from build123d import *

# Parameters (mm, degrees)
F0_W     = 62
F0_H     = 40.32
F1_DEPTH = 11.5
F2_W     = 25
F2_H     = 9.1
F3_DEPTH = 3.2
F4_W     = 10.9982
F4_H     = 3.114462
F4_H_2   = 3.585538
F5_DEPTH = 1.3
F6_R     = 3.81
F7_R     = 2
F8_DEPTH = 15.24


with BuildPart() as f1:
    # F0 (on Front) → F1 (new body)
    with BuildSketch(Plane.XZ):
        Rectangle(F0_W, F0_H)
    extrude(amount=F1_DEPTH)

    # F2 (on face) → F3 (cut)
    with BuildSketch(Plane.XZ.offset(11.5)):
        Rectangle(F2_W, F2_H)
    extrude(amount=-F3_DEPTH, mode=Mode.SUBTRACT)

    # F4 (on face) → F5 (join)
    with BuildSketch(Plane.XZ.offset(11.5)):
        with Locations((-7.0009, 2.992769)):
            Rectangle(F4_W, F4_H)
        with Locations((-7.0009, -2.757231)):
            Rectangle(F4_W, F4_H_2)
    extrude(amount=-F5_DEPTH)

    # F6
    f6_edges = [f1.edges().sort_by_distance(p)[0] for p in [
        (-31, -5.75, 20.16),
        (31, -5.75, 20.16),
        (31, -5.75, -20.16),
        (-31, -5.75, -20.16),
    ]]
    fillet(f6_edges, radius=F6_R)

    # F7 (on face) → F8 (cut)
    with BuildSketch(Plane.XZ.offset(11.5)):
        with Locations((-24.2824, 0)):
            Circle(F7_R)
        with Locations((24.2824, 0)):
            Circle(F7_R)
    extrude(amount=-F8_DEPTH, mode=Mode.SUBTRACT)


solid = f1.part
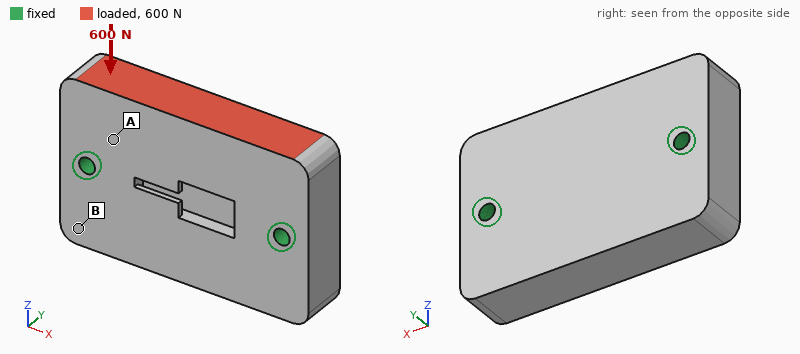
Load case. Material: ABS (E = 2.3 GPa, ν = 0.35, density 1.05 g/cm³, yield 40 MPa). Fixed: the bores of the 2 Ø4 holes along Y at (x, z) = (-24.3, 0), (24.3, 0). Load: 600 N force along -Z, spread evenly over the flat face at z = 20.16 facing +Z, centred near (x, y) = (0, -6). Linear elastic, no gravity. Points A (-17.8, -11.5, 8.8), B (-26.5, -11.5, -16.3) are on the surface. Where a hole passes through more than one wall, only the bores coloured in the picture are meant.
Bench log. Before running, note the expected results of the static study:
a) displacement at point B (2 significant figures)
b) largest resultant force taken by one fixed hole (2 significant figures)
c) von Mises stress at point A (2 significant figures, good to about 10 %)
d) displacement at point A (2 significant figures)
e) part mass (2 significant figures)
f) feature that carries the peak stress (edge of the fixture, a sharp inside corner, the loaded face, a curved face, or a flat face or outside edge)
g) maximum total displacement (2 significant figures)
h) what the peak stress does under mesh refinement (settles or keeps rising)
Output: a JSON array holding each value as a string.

["4.9 µm", "300 N", "1.5 MPa", "11 µm", "29 g", "edge of the fixture", "23 µm", "keeps rising"]
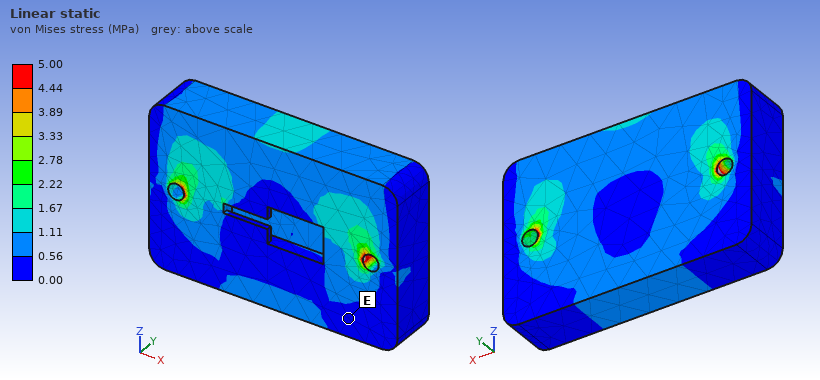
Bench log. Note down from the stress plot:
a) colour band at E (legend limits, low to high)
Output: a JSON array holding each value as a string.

["0.00 to 0.56 MPa"]
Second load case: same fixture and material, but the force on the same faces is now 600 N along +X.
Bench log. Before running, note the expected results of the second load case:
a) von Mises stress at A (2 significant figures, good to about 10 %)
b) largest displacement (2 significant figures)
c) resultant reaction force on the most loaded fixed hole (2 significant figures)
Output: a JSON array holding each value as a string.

["1.9 MPa", "37 µm", "380 N"]
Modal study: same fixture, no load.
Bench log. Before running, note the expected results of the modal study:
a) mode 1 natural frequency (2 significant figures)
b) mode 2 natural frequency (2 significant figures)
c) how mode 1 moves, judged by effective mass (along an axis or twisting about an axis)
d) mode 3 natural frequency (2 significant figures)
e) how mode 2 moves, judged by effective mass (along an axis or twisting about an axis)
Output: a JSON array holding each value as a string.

["3200 Hz", "3700 Hz", "twisting about X", "5700 Hz", "along Y"]
